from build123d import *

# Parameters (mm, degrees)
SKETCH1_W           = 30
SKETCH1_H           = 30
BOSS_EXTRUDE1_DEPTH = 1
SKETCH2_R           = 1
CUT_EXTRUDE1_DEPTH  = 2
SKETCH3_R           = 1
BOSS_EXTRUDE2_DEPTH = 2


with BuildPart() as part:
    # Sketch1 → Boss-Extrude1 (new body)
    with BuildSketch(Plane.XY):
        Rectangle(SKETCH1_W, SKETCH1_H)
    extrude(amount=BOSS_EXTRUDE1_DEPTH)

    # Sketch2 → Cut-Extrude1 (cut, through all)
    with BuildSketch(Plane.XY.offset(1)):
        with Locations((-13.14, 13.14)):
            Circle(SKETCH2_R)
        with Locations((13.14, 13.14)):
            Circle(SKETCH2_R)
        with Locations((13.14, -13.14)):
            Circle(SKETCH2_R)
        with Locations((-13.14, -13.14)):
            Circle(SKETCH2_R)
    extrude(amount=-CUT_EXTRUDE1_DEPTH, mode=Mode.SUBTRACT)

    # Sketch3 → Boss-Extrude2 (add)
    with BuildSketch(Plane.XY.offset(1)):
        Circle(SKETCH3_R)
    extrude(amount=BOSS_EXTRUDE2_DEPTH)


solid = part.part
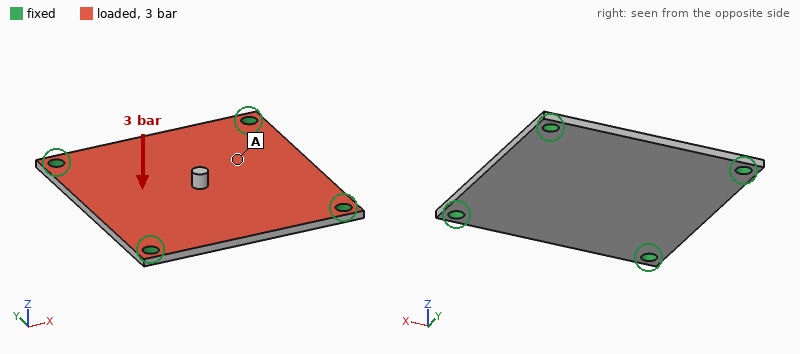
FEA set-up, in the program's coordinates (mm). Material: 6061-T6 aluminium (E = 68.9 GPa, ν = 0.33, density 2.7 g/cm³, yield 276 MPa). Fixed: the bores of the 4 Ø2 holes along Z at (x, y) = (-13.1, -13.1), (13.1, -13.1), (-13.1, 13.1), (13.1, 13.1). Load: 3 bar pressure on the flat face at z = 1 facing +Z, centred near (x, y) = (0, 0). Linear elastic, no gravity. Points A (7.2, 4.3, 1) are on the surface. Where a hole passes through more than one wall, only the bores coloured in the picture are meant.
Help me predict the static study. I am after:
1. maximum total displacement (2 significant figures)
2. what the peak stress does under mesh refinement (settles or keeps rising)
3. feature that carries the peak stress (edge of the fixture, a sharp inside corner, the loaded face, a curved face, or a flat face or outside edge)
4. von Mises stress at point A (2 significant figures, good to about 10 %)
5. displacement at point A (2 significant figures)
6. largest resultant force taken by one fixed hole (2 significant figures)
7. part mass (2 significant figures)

0.15 mm
keeps rising
edge of the fixture
47 MPa
0.11 mm
66 N
2.4 g
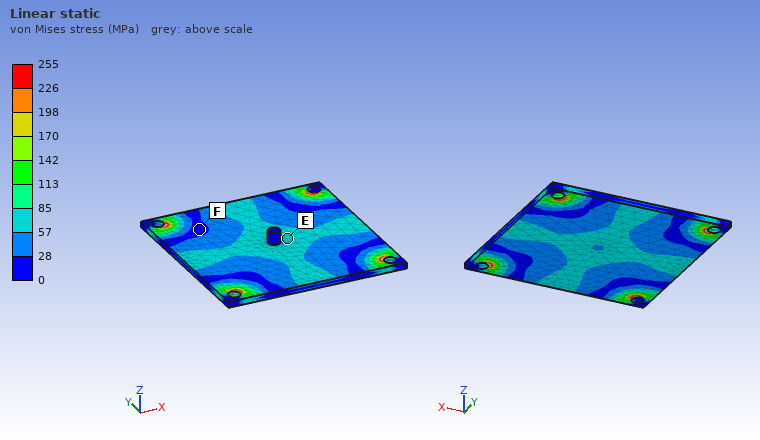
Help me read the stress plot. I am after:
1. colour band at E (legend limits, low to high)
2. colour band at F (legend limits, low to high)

57 to 85 MPa
0 to 28 MPa
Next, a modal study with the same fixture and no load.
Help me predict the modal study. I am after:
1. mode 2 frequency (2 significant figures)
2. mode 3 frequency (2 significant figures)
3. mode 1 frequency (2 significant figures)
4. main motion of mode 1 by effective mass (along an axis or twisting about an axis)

8900 Hz
8900 Hz
5100 Hz
along Z
